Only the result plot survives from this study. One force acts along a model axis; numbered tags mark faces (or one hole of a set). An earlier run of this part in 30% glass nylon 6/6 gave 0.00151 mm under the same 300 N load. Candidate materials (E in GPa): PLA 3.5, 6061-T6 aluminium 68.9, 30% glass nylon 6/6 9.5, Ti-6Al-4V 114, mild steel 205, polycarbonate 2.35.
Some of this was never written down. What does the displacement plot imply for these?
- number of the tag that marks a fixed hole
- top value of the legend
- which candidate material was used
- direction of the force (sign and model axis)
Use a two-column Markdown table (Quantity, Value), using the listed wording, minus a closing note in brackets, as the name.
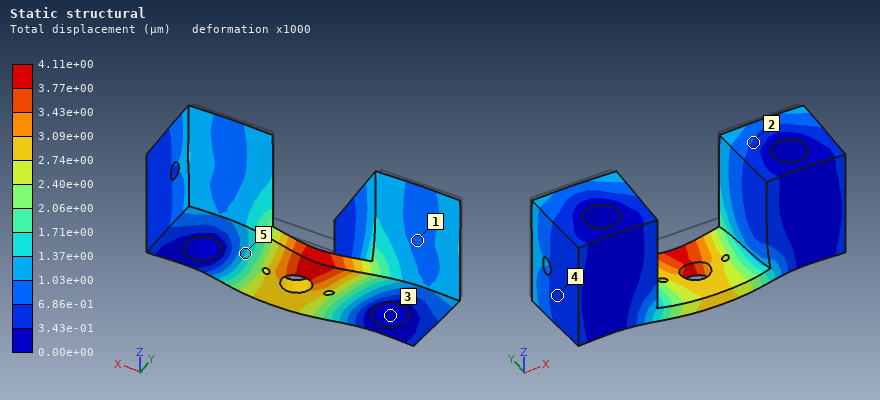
| Quantity | Value |
|---|---|
| number of the tag that marks a fixed hole | 3 |
| top value of the legend | 4.11e+00 µm |
| which candidate material was used | PLA |
| direction of the force | -Y |
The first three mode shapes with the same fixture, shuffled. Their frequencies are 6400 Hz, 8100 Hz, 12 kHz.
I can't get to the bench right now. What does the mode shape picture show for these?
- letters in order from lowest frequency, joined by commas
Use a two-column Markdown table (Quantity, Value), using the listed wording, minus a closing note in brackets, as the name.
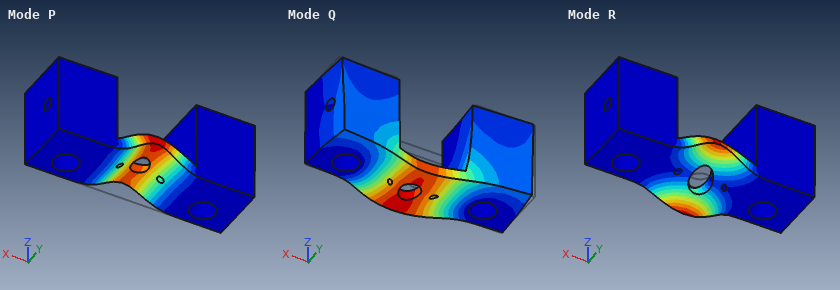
| Quantity | Value |
|---|---|
| letters in order from lowest frequency, joined by commas | P, R, Q |
